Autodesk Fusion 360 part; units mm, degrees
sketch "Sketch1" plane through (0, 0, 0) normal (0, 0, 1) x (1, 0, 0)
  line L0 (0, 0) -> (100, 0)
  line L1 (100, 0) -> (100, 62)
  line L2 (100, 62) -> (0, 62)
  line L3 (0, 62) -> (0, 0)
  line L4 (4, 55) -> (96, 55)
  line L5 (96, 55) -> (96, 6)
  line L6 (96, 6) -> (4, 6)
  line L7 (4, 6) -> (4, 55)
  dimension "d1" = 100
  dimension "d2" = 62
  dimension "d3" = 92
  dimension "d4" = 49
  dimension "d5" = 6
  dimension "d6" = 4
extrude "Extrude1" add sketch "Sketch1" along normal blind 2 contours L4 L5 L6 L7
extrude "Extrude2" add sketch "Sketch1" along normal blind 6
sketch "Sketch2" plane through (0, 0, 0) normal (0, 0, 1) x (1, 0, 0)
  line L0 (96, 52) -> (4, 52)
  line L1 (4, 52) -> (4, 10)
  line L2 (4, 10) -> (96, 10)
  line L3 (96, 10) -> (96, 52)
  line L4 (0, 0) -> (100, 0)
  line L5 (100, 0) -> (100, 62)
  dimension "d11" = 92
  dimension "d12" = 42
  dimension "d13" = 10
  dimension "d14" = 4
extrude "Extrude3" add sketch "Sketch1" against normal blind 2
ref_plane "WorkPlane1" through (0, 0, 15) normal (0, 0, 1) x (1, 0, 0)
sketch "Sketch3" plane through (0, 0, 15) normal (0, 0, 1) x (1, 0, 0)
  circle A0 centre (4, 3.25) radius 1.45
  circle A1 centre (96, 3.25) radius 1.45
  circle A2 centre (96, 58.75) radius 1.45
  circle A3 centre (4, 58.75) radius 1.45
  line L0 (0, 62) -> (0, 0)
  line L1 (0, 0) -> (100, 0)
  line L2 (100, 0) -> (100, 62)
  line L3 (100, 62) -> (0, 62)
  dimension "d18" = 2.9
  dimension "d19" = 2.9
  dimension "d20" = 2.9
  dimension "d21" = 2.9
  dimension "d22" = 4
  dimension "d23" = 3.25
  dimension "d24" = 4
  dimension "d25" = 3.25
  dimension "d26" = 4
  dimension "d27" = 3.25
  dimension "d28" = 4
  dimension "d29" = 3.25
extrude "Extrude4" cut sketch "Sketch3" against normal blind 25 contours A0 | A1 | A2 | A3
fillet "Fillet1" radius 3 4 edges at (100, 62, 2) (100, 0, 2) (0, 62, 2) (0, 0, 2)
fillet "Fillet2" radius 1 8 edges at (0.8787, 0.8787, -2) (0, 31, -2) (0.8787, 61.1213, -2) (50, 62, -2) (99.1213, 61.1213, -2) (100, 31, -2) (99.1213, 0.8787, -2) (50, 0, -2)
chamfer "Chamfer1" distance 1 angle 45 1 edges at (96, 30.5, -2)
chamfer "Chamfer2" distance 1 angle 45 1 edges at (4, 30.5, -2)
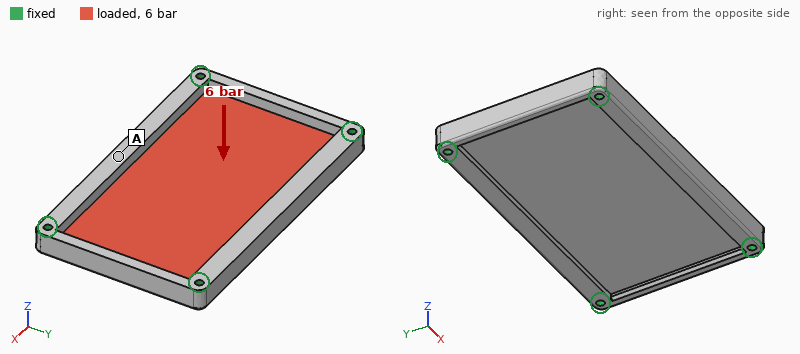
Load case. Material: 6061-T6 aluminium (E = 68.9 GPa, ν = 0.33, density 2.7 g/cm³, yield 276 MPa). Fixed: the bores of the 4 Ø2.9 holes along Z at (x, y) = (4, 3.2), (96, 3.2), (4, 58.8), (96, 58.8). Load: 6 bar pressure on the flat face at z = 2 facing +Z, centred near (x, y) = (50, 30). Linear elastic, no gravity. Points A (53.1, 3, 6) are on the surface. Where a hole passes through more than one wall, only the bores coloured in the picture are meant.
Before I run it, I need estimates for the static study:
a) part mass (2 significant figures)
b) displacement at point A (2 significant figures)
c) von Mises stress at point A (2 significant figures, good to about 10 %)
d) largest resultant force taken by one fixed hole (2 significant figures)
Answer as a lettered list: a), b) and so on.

a) 60 g
b) 0.15 mm
c) 70 MPa
d) 710 N
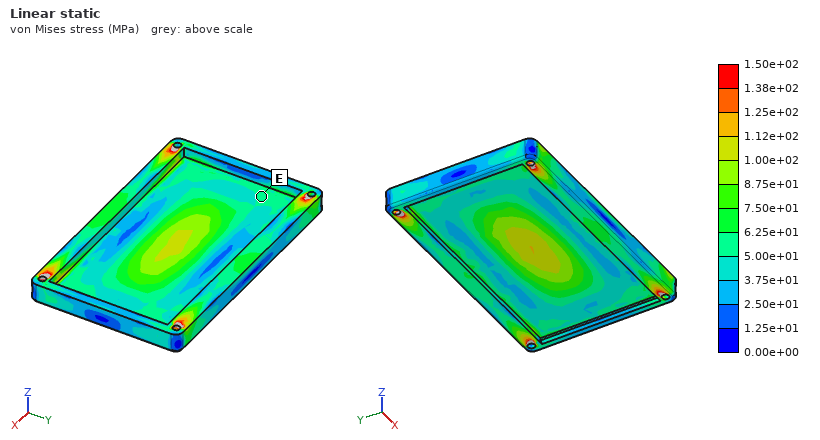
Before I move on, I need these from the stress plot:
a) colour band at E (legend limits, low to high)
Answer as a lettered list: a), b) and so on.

a) 5.00e+01 to 6.25e+01 MPa
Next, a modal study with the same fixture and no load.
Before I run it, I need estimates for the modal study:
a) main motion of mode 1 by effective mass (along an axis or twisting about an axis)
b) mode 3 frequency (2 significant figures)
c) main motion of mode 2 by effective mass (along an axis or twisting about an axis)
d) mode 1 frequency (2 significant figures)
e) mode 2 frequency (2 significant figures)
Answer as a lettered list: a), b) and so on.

a) along Z
b) 5300 Hz
c) twisting about X
d) 2900 Hz
e) 4300 Hz
